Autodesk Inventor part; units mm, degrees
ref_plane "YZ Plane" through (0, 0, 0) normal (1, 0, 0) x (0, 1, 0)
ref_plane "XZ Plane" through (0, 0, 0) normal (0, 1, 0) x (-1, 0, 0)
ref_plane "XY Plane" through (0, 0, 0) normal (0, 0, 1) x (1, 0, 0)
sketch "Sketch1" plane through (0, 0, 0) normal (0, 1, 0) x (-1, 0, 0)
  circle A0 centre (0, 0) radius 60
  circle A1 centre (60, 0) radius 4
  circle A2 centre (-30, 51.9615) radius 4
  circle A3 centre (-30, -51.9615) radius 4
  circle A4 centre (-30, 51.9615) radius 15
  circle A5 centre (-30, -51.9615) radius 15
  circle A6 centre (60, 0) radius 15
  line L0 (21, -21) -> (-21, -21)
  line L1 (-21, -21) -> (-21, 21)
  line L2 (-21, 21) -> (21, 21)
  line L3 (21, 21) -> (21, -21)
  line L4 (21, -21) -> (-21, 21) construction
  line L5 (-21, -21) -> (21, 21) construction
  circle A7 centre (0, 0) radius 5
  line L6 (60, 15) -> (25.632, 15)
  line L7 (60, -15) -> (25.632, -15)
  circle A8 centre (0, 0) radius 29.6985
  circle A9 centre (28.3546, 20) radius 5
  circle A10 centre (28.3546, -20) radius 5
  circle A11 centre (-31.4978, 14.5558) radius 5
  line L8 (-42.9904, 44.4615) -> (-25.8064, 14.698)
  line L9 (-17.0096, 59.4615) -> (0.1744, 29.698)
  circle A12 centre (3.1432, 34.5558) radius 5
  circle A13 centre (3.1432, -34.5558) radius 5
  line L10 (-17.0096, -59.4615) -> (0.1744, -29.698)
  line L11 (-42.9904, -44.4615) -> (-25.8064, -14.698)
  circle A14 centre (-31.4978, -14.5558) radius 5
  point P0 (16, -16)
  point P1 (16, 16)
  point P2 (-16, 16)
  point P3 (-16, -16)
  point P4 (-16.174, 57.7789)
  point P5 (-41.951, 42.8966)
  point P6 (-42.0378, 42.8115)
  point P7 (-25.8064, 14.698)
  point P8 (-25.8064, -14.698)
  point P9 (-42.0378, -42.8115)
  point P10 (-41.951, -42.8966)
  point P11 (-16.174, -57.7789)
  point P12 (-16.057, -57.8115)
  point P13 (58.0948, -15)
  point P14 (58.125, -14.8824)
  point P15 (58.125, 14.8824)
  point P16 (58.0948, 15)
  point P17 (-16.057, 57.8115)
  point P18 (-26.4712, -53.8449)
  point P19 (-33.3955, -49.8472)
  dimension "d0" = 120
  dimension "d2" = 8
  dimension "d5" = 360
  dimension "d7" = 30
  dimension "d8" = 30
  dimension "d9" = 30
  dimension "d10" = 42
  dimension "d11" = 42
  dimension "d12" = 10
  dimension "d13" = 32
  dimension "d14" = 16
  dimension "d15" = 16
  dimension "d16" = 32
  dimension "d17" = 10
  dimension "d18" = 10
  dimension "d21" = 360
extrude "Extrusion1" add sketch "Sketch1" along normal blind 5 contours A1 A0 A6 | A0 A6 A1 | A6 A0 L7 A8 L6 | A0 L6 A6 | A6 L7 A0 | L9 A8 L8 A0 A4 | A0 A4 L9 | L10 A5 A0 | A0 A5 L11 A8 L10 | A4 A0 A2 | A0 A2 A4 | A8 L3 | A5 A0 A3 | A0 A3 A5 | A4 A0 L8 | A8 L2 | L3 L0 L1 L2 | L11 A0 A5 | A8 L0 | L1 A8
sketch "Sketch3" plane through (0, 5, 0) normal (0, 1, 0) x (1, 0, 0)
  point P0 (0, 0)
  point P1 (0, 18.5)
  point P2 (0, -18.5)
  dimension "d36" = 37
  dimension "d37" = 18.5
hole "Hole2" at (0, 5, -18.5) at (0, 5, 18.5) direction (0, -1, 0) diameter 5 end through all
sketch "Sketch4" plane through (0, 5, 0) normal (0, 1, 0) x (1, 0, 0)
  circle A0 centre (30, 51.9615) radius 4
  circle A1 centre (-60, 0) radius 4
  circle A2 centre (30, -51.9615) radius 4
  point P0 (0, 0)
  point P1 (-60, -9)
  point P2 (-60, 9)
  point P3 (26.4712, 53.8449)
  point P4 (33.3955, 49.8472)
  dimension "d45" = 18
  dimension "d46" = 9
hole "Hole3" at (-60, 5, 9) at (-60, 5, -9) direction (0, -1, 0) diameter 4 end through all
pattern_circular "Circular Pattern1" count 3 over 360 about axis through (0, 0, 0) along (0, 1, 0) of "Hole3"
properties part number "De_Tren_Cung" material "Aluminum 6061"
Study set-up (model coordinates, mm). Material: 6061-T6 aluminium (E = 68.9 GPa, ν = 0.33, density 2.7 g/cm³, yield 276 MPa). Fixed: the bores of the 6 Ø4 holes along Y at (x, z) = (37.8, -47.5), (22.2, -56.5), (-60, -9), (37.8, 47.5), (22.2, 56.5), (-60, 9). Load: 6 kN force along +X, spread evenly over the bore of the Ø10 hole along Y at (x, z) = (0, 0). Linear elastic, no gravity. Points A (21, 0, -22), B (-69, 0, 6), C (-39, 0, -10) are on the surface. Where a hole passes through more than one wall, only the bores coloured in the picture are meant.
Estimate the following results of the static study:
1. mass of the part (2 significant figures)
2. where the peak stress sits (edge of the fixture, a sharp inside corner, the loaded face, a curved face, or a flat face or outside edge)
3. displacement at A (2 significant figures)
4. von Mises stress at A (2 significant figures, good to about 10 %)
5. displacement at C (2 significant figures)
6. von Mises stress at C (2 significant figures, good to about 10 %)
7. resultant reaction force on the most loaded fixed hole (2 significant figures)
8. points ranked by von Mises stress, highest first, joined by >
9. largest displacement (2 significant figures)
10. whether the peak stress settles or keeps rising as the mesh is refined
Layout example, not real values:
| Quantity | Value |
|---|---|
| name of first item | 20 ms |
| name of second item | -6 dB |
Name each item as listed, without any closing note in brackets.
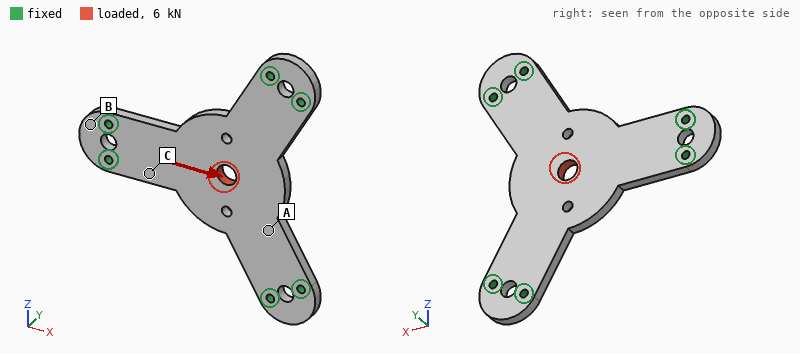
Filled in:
| Quantity | Value |
|---|---|
| mass of the part | 85 g |
| where the peak stress sits | edge of the fixture |
| displacement at A | 14 µm |
| von Mises stress at A | 14 MPa |
| displacement at C | 7.7 µm |
| von Mises stress at C | 23 MPa |
| resultant reaction force on the most loaded fixed hole | 1.7 kN |
| points ranked by von Mises stress, highest first, joined by > | C > A > B |
| largest displacement | 27 µm |
| whether the peak stress settles or keeps rising as the mesh is refined | keeps rising |
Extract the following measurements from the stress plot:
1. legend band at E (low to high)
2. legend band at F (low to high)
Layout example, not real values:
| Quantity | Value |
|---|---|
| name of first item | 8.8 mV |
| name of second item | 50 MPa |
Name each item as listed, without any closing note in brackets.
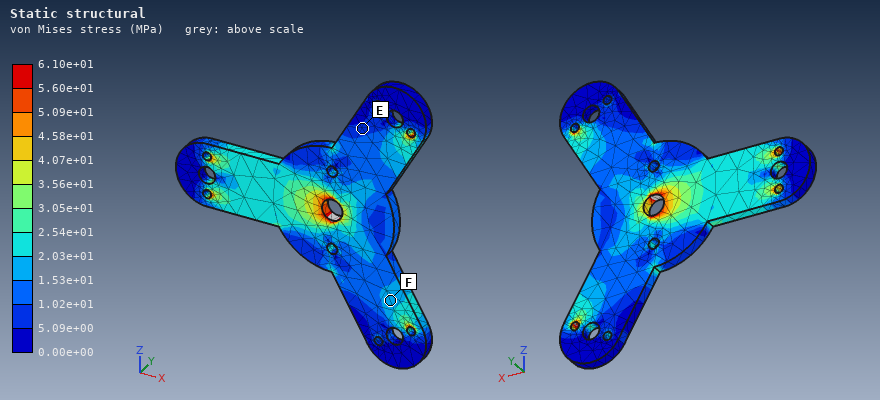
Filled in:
| Quantity | Value |
|---|---|
| legend band at E | 5.09e+00 to 1.02e+01 MPa |
| legend band at F | 1.53e+01 to 2.03e+01 MPa |
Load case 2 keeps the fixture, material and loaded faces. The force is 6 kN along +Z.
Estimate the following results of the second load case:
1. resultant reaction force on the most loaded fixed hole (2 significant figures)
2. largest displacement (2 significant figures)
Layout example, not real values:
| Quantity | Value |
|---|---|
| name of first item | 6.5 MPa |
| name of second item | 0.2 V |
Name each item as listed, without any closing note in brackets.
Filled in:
| Quantity | Value |
|---|---|
| resultant reaction force on the most loaded fixed hole | 1.9 kN |
| largest displacement | 28 µm |
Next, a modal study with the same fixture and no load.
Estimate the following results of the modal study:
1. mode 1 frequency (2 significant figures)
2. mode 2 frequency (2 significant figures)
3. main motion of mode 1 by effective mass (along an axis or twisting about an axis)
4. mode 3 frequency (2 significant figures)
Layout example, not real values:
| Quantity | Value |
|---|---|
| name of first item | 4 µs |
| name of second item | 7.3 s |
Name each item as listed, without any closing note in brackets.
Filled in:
| Quantity | Value |
|---|---|
| mode 1 frequency | 2000 Hz |
| mode 2 frequency | 4300 Hz |
| main motion of mode 1 by effective mass | along Y |
| mode 3 frequency | 4400 Hz |
